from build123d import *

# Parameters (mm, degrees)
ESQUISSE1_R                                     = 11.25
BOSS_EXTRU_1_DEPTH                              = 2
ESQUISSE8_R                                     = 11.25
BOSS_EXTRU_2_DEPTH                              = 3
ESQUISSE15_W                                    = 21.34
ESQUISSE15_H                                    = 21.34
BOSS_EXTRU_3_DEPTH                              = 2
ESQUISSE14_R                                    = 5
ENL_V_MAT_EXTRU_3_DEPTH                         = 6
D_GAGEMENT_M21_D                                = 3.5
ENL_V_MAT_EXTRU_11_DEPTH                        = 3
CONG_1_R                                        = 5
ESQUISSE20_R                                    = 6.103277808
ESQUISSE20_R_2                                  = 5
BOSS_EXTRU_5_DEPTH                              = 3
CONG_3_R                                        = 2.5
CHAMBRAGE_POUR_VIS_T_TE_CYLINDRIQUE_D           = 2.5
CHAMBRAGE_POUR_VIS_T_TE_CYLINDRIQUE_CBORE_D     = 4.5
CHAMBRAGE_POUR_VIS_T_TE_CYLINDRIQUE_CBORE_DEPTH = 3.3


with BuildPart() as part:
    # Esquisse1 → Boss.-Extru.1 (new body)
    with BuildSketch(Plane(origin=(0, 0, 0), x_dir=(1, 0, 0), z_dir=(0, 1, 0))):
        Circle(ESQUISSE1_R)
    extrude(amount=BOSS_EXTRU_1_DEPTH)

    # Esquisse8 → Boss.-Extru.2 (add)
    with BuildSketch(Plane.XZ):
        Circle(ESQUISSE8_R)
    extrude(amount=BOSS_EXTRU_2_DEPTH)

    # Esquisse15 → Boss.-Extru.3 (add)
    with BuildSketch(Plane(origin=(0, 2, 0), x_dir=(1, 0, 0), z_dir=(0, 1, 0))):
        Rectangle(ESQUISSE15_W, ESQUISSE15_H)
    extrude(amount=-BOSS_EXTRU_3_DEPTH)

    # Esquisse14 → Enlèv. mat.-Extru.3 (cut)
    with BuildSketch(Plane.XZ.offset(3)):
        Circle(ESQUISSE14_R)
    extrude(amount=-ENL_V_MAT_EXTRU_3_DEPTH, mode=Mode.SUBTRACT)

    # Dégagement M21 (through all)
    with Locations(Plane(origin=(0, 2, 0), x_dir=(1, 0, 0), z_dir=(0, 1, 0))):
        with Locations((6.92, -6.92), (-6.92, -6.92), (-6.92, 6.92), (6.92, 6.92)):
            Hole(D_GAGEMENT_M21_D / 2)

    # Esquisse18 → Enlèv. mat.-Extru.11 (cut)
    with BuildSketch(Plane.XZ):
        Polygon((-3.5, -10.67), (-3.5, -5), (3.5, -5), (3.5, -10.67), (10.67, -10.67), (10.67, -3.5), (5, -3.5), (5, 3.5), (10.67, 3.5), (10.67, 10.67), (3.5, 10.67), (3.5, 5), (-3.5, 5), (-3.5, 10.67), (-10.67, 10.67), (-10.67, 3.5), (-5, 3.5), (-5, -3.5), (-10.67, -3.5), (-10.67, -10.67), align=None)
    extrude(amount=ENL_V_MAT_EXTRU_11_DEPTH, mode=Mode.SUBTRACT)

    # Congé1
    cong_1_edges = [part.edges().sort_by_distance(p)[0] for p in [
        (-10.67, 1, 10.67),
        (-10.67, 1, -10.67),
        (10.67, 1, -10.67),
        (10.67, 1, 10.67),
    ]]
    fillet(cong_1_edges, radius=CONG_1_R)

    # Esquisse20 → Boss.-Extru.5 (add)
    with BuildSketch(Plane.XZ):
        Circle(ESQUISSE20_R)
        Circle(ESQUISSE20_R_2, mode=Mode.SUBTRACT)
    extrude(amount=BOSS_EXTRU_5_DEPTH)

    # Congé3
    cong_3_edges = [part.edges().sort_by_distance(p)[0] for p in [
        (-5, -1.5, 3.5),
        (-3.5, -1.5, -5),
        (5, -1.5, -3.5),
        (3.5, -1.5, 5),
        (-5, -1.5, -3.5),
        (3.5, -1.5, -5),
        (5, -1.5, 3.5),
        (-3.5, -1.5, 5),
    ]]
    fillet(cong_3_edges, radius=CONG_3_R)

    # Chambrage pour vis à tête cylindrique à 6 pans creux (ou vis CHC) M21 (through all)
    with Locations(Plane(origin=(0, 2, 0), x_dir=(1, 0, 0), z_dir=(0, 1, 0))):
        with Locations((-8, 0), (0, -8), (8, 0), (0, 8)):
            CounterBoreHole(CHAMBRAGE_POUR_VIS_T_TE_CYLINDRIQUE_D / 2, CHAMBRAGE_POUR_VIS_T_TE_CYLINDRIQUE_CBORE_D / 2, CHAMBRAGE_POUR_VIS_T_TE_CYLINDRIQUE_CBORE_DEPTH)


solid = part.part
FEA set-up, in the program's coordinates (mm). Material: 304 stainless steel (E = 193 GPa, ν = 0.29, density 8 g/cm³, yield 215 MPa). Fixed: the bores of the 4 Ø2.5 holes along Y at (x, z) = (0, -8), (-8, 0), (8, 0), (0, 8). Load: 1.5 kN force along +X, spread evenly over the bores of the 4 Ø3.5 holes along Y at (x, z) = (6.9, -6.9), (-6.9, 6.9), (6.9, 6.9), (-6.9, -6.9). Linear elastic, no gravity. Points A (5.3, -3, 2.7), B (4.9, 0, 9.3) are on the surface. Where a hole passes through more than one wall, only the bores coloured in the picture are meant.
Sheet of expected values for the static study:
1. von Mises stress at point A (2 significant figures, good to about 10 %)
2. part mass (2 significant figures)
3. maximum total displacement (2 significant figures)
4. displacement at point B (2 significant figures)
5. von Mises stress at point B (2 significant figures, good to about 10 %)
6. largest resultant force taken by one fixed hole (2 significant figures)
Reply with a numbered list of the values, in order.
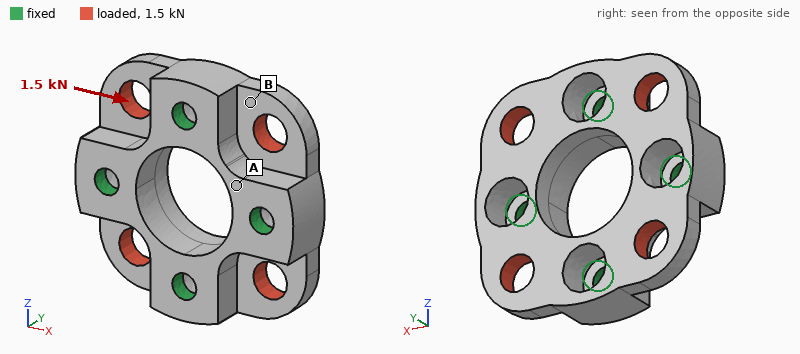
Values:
1. 21 MPa
2. 7.8 g
3. 5.0 µm
4. 3.4 µm
5. 49 MPa
6. 440 N
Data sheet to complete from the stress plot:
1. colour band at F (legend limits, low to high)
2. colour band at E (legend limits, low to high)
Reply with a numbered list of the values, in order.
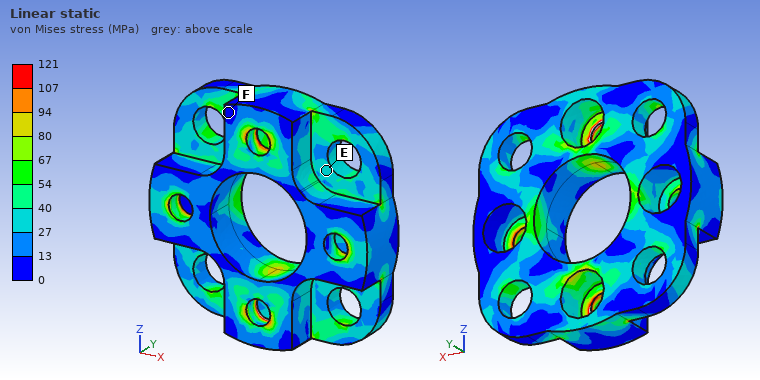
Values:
1. 0 to 13 MPa
2. 27 to 40 MPa
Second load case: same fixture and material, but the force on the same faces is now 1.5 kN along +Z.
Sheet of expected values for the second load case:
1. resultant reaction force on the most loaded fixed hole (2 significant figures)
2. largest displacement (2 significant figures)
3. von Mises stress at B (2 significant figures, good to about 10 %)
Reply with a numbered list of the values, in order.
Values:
1. 440 N
2. 5.0 µm
3. 30 MPa
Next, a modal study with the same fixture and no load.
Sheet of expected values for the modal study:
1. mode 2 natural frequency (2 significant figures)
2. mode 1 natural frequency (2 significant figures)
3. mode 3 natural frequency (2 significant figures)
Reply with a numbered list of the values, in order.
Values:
1. 41 kHz
2. 36 kHz
3. 41 kHz
